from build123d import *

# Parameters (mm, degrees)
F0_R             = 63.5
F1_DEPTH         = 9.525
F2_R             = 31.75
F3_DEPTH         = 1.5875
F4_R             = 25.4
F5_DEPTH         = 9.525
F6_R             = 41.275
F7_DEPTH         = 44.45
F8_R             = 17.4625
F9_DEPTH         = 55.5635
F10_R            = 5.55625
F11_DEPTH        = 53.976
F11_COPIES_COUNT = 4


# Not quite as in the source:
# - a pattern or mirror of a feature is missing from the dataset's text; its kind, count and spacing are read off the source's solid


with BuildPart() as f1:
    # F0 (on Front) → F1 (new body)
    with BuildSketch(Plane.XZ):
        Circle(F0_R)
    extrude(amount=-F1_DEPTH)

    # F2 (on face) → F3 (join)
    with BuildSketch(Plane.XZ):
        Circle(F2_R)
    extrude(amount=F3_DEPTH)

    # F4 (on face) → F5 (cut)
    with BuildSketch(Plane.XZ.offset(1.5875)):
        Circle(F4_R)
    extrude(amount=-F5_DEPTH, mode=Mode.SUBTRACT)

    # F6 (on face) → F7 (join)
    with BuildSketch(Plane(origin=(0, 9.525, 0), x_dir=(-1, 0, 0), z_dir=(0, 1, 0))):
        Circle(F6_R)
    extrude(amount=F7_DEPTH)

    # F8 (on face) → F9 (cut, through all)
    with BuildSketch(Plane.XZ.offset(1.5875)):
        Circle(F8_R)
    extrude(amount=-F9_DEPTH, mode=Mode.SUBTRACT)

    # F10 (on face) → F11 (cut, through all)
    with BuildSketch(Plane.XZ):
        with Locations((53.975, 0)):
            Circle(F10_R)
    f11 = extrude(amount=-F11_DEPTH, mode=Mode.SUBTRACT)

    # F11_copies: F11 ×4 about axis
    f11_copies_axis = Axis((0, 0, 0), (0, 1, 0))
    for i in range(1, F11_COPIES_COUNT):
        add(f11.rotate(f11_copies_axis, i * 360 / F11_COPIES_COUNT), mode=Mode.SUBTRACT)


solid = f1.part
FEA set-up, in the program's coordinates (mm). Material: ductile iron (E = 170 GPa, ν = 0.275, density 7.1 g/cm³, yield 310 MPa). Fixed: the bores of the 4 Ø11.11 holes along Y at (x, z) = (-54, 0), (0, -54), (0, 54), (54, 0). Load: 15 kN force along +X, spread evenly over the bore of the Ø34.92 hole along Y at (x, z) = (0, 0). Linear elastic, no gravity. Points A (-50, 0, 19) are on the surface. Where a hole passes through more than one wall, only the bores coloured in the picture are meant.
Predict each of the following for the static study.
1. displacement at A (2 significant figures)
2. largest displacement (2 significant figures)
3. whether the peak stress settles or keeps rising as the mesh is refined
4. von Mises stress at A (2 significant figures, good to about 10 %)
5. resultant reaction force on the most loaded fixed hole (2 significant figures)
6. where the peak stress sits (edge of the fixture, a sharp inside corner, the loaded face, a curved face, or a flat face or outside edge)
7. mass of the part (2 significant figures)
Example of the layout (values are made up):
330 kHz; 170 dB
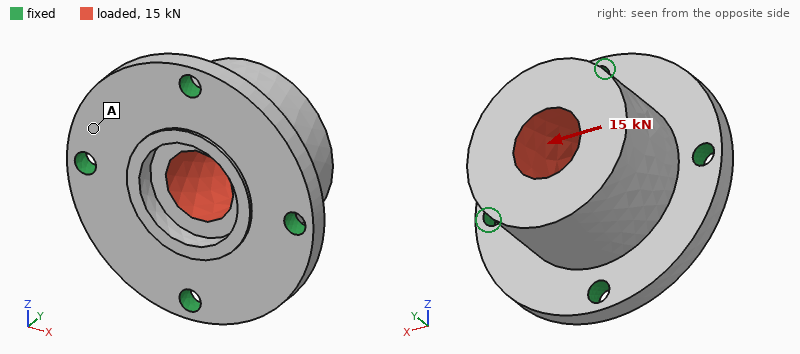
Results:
3.4 µm; 11 µm; keeps rising; 7.0 MPa; 6.3 kN; edge of the fixture; 2.1 kg
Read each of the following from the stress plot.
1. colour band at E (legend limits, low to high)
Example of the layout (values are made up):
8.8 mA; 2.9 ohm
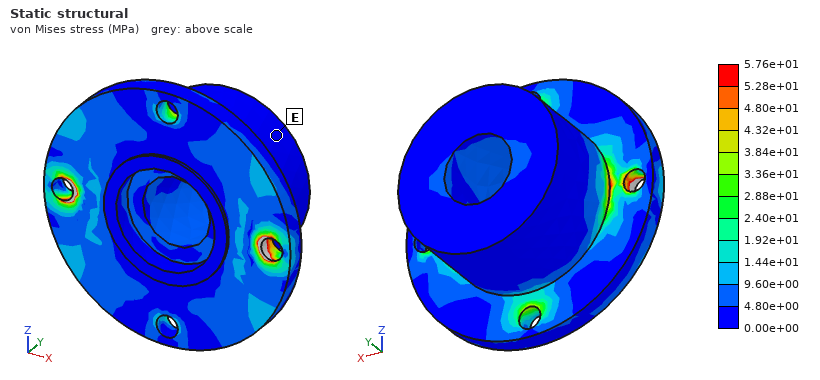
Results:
0.00e+00 to 4.80e+00 MPa
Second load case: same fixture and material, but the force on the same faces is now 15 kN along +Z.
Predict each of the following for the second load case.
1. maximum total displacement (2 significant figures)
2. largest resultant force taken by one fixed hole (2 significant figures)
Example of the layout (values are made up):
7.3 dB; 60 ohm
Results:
11 µm; 6.3 kN
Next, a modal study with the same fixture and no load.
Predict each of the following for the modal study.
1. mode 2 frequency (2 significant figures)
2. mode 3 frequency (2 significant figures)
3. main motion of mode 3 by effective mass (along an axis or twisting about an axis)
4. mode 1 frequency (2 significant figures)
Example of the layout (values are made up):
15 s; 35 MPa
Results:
5100 Hz; 5700 Hz; along Y; 5100 Hz
